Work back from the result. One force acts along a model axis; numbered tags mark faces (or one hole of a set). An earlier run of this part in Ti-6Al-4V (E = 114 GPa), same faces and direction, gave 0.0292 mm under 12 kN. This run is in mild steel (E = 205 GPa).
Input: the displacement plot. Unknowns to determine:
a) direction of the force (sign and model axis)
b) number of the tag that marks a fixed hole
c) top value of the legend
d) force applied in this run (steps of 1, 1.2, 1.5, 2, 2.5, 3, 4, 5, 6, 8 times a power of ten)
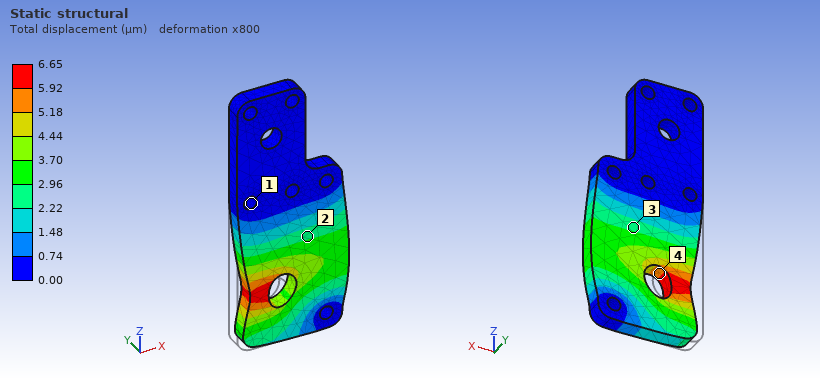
+X
1
6.65 µm
5 kN
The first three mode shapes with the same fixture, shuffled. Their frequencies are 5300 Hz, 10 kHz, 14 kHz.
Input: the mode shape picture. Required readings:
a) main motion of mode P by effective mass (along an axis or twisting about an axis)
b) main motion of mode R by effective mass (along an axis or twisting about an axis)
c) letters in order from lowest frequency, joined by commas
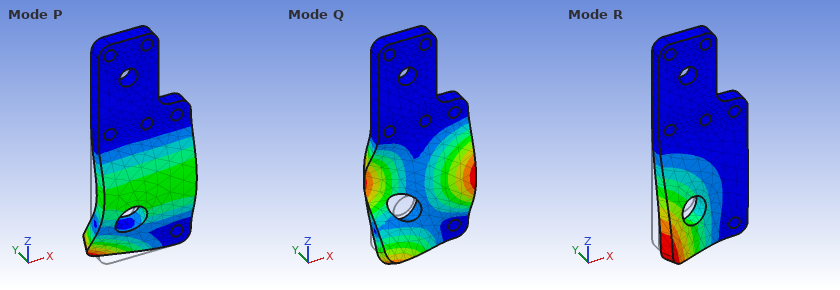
along Y
along Y
R, P, Q
